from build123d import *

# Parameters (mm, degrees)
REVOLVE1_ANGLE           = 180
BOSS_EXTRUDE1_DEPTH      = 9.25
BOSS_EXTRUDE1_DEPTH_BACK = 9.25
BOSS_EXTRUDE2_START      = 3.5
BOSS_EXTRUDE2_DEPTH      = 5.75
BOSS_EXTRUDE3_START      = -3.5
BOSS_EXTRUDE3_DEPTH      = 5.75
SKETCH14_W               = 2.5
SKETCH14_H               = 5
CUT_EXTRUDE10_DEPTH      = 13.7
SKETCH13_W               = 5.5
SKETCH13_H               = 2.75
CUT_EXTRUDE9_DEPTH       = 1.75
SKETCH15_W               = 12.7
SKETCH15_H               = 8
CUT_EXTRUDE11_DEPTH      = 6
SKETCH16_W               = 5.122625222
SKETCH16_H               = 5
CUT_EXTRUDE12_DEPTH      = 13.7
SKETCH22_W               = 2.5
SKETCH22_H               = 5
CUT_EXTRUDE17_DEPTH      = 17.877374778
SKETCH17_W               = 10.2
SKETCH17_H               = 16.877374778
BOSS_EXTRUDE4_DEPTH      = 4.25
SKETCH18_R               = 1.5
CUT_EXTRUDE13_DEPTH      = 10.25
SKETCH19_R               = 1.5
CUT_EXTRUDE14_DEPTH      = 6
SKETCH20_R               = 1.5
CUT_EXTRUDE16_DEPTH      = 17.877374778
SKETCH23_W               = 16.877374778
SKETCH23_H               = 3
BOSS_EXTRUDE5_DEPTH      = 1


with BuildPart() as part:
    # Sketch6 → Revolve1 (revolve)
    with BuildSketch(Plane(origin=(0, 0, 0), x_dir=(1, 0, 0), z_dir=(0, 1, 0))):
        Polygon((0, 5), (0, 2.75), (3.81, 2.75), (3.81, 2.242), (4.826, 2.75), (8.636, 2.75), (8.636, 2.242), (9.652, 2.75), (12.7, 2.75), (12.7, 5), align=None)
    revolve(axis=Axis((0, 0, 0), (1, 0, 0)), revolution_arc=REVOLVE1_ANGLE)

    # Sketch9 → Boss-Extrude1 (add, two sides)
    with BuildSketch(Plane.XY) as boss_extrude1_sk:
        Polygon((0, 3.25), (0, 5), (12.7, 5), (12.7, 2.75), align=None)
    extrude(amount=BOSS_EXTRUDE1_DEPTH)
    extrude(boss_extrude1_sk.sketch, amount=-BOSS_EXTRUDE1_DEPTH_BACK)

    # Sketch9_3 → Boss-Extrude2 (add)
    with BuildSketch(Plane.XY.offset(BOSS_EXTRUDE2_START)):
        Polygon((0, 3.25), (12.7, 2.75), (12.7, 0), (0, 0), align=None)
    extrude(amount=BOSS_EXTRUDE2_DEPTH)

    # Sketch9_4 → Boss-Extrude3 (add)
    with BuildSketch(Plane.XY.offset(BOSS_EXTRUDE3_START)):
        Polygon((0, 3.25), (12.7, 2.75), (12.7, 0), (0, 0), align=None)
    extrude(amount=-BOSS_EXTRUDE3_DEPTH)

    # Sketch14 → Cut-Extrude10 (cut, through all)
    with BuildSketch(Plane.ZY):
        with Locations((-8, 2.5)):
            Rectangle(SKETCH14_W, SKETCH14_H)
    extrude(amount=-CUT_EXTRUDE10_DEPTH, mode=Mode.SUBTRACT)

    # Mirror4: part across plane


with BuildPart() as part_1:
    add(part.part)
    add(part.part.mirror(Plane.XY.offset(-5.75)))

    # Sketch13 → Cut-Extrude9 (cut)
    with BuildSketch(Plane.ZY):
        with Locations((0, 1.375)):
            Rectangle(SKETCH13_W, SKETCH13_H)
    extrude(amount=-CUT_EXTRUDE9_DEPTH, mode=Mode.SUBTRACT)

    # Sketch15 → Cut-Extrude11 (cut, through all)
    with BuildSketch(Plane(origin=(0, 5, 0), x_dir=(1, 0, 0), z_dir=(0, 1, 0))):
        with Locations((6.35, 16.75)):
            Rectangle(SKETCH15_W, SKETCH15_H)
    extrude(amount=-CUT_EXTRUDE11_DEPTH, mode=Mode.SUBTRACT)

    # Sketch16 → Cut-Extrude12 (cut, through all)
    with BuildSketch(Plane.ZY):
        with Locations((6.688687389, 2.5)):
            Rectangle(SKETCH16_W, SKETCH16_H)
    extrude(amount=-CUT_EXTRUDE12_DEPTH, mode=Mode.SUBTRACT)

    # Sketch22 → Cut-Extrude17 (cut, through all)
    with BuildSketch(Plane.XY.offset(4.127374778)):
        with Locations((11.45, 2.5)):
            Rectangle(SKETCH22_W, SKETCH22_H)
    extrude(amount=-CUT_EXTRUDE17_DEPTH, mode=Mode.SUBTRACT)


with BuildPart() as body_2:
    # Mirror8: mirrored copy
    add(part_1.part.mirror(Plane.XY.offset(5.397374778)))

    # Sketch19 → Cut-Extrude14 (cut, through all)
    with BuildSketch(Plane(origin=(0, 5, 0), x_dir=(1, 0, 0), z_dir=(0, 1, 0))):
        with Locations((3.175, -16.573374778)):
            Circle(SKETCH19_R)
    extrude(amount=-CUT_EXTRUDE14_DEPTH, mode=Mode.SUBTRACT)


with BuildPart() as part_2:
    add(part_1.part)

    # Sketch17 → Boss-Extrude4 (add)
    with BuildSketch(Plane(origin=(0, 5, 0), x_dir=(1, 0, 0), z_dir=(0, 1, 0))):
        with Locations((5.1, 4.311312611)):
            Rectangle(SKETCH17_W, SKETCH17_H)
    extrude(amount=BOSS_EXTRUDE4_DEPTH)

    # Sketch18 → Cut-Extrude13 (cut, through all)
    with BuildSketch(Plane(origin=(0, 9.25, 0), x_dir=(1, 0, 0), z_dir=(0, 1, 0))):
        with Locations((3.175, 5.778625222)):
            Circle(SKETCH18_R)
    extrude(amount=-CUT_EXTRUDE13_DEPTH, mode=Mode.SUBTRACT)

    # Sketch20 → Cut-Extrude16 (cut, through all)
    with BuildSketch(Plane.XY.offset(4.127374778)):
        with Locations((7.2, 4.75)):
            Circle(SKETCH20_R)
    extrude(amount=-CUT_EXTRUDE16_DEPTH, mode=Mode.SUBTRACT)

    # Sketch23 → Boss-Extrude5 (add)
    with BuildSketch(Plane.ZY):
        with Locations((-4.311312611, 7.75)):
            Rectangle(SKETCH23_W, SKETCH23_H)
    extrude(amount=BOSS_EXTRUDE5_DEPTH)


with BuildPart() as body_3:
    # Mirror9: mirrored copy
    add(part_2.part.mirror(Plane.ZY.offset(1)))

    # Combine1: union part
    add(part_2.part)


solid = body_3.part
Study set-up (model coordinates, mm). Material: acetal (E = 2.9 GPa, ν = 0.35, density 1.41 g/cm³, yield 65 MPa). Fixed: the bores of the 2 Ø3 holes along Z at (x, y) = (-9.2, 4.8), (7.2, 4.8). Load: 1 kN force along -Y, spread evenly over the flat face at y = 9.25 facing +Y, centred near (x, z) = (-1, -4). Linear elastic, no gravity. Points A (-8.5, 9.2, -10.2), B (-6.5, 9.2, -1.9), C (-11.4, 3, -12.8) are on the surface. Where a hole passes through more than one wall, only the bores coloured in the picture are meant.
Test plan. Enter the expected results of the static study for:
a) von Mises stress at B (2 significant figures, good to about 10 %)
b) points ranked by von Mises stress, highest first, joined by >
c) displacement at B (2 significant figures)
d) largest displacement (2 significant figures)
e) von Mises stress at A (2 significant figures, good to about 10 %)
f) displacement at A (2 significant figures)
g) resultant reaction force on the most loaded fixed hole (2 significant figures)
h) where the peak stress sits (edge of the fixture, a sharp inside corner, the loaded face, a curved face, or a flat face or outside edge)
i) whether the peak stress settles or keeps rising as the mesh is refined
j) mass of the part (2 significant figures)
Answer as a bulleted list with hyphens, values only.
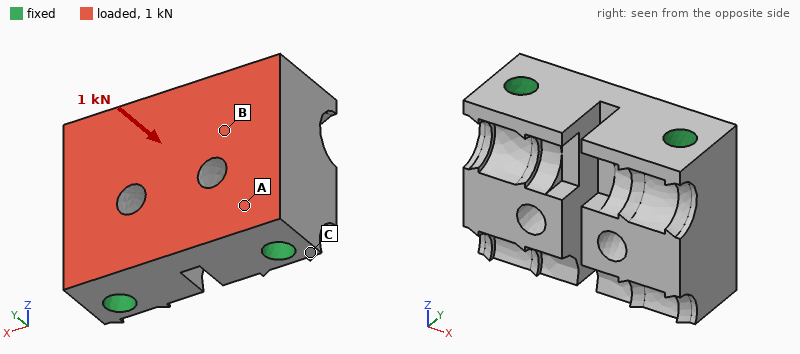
- 2.7 MPa
- A > B > C
- 11 µm
- 25 µm
- 5.0 MPa
- 6.8 µm
- 530 N
- edge of the fixture
- keeps rising
- 3.5 g
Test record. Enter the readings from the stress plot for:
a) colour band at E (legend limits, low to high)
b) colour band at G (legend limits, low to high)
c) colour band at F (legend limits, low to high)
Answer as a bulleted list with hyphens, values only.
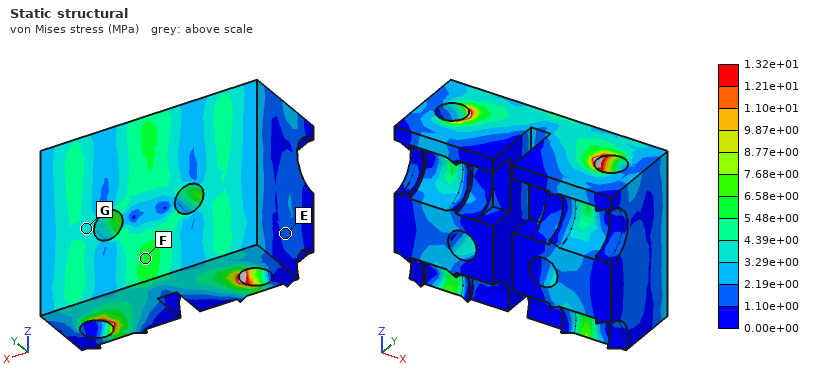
- 1.10e+00 to 2.19e+00 MPa
- 3.29e+00 to 4.39e+00 MPa
- 5.48e+00 to 6.58e+00 MPa
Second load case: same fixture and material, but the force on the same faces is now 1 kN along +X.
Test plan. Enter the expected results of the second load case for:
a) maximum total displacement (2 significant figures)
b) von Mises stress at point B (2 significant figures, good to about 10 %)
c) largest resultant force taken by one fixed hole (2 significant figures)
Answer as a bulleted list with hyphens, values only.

- 23 µm
- 4.9 MPa
- 530 N
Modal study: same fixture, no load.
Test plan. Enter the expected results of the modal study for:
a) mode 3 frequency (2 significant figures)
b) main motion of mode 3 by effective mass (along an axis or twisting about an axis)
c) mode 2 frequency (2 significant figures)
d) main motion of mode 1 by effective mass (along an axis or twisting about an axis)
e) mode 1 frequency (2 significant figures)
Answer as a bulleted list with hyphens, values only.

- 26 kHz
- along Z
- 24 kHz
- along Y
- 20 kHz
